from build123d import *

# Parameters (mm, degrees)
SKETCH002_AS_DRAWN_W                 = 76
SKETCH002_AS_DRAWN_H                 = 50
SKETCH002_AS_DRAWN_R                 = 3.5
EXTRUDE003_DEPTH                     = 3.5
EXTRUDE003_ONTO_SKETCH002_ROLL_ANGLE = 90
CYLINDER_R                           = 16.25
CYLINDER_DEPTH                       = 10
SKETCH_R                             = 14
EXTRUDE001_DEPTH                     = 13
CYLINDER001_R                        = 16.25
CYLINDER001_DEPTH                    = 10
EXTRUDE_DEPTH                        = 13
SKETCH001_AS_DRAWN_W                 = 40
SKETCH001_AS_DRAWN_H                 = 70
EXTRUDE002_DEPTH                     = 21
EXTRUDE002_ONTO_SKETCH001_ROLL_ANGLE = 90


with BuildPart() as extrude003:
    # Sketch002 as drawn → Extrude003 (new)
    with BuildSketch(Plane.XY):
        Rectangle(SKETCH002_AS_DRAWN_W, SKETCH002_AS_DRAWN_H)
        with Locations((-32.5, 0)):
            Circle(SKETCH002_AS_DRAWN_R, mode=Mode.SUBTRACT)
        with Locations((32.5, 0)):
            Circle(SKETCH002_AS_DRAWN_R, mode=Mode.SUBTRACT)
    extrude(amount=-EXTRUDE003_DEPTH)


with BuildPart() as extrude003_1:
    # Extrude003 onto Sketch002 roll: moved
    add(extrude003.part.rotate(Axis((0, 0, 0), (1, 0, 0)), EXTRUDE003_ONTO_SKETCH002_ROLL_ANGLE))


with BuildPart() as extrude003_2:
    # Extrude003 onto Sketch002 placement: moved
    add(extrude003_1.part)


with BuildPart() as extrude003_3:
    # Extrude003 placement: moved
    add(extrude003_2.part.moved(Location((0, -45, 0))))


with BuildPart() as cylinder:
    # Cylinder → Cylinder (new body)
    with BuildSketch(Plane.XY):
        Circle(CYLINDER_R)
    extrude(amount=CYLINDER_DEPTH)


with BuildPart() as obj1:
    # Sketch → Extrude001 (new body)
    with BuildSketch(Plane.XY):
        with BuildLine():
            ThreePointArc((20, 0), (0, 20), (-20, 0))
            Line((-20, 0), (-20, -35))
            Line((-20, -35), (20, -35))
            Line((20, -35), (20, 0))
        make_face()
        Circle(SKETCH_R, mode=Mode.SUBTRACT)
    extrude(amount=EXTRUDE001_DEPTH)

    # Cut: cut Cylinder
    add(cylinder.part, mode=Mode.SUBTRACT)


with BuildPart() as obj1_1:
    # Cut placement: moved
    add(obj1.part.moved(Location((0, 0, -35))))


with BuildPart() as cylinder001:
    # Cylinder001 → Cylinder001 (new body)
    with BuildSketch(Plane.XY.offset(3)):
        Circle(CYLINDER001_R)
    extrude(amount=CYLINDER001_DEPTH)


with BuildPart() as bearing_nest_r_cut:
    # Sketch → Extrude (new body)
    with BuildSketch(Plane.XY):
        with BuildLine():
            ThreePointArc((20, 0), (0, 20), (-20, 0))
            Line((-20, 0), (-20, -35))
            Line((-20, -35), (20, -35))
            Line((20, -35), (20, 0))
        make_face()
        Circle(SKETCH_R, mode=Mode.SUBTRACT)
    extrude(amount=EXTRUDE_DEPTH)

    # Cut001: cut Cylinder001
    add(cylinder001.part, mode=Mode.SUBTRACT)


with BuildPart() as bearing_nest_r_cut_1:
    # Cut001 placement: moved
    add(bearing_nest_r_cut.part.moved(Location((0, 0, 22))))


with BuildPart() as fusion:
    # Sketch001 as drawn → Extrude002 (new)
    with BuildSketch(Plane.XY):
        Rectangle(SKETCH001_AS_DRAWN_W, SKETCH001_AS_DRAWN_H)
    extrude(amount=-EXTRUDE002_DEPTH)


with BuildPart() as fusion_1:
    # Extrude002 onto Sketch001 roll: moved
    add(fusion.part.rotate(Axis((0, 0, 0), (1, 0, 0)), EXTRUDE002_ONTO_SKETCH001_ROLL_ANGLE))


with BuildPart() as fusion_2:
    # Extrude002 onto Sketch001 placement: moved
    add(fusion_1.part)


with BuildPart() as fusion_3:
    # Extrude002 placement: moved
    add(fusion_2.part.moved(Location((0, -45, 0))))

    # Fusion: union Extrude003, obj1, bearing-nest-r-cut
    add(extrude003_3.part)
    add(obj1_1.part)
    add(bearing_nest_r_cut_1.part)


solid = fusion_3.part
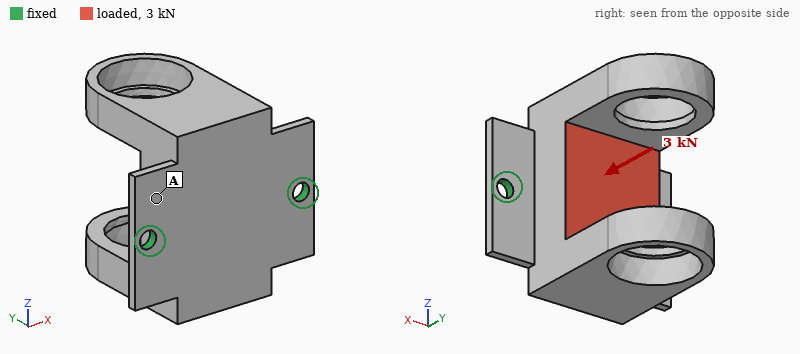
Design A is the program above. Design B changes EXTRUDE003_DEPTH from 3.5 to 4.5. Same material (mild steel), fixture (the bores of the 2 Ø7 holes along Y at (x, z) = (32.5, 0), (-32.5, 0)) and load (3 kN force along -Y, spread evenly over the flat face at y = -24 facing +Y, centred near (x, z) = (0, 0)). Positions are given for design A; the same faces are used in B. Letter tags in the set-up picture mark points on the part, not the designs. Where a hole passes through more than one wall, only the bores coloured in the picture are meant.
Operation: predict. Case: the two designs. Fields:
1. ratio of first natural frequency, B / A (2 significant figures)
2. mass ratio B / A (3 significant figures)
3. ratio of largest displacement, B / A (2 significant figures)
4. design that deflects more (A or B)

1.4
1.02
0.62
A
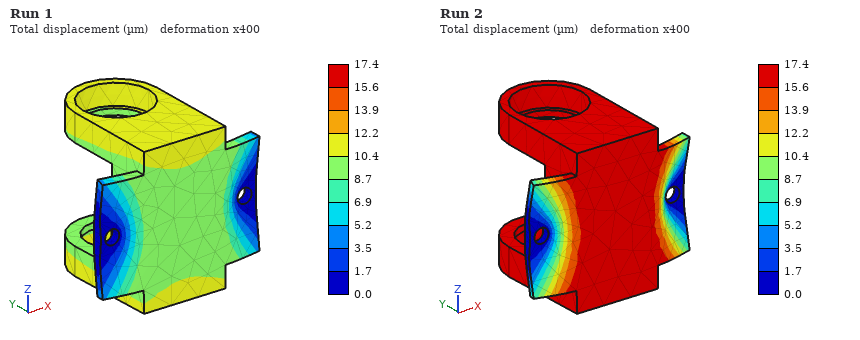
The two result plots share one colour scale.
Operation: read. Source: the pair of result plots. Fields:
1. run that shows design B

Run 1
